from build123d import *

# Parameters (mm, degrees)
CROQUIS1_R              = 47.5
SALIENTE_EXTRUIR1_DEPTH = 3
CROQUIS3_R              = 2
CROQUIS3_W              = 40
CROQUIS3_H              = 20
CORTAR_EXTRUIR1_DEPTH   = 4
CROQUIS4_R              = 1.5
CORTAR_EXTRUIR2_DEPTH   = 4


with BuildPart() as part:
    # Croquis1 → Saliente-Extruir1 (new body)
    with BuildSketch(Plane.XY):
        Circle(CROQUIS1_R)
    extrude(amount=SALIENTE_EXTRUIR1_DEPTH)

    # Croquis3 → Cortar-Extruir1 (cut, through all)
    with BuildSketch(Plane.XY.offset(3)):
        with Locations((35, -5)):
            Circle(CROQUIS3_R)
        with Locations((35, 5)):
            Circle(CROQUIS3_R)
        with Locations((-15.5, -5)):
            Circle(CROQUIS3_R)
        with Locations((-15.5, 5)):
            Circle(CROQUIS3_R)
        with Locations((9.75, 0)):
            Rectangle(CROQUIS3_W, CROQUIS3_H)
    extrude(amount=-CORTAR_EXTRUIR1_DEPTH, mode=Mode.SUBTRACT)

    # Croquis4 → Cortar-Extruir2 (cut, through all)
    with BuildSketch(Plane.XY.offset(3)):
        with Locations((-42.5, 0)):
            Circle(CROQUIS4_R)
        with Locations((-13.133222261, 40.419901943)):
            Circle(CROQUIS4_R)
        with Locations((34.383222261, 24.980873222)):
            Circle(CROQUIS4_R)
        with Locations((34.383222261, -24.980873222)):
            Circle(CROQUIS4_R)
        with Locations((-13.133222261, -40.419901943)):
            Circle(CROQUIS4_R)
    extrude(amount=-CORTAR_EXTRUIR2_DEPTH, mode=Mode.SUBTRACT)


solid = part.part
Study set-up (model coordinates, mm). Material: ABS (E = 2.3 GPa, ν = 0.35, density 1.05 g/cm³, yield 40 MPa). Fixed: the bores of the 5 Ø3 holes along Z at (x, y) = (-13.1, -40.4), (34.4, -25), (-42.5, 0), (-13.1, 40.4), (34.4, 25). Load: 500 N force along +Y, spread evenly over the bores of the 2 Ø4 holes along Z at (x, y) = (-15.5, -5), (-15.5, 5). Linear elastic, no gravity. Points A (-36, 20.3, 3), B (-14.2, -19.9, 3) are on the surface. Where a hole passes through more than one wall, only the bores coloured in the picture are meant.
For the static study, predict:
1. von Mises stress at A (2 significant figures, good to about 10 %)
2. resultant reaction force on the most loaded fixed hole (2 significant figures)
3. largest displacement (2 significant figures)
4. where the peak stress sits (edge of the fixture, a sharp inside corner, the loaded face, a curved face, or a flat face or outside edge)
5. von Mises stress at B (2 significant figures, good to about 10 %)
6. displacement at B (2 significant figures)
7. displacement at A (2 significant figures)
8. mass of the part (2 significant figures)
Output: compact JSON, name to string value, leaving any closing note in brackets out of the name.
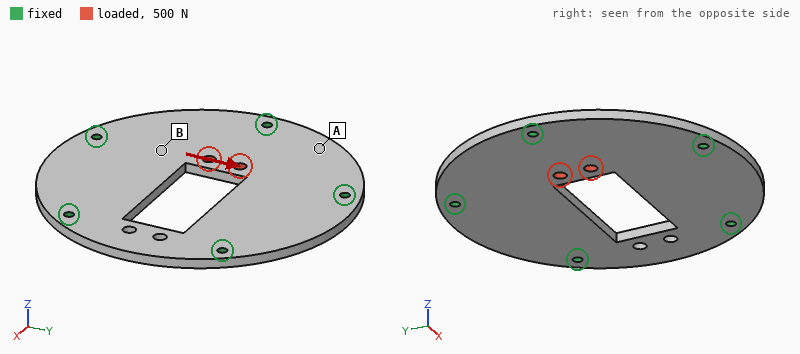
{"von Mises stress at A": "1.6 MPa", "resultant reaction force on the most loaded fixed hole": "170 N", "largest displacement": "91 µm", "where the peak stress sits": "the loaded face", "von Mises stress at B": "4.6 MPa", "displacement at B": "43 µm", "displacement at A": "36 µm", "mass of the part": "20 g"}
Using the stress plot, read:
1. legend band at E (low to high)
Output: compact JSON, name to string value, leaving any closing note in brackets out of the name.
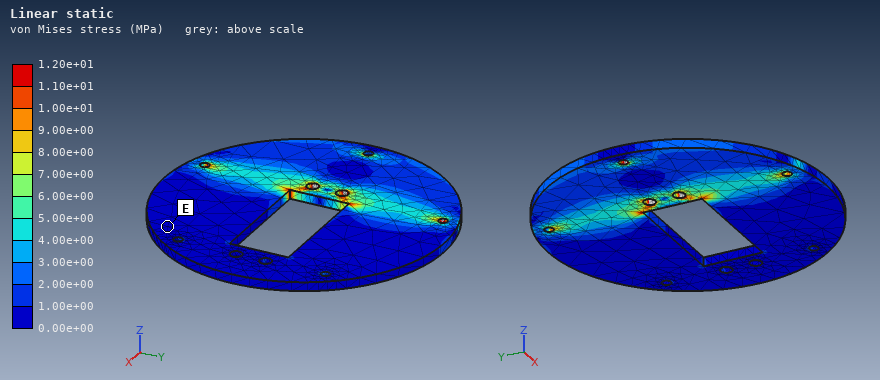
{"legend band at E": "0.00e+00 to 1.00e+00 MPa"}
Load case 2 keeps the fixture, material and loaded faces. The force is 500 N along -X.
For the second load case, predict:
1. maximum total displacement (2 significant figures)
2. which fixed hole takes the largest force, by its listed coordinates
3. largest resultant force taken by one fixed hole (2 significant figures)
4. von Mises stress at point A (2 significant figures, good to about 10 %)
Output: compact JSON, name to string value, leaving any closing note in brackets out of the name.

{"maximum total displacement": "93 µm", "which fixed hole takes the largest force, by its listed coordinates": "(-42.5, 0)", "largest resultant force taken by one fixed hole": "260 N", "von Mises stress at point A": "1.3 MPa"}
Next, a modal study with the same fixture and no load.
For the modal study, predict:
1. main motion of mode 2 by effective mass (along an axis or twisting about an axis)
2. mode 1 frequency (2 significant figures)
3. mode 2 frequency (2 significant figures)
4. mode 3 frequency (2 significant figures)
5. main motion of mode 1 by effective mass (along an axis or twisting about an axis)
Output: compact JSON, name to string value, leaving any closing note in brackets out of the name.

{"main motion of mode 2 by effective mass": "twisting about X", "mode 1 frequency": "980 Hz", "mode 2 frequency": "1400 Hz", "mode 3 frequency": "1500 Hz", "main motion of mode 1 by effective mass": "along Z"}
